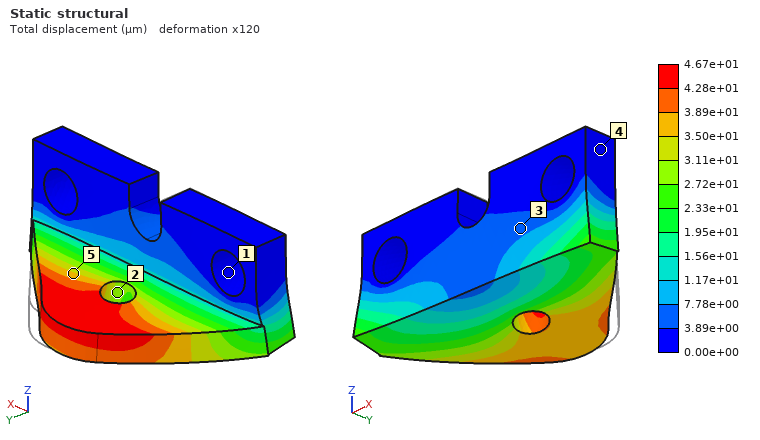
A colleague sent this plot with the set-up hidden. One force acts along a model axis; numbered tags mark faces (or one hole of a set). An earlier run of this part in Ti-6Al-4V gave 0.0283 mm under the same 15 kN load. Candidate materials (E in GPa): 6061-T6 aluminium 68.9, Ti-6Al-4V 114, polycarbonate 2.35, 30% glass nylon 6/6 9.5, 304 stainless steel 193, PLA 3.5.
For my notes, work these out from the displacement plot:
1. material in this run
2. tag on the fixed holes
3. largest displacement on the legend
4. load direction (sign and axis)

6061-T6 aluminium
1
4.67e+01 µm
-X
